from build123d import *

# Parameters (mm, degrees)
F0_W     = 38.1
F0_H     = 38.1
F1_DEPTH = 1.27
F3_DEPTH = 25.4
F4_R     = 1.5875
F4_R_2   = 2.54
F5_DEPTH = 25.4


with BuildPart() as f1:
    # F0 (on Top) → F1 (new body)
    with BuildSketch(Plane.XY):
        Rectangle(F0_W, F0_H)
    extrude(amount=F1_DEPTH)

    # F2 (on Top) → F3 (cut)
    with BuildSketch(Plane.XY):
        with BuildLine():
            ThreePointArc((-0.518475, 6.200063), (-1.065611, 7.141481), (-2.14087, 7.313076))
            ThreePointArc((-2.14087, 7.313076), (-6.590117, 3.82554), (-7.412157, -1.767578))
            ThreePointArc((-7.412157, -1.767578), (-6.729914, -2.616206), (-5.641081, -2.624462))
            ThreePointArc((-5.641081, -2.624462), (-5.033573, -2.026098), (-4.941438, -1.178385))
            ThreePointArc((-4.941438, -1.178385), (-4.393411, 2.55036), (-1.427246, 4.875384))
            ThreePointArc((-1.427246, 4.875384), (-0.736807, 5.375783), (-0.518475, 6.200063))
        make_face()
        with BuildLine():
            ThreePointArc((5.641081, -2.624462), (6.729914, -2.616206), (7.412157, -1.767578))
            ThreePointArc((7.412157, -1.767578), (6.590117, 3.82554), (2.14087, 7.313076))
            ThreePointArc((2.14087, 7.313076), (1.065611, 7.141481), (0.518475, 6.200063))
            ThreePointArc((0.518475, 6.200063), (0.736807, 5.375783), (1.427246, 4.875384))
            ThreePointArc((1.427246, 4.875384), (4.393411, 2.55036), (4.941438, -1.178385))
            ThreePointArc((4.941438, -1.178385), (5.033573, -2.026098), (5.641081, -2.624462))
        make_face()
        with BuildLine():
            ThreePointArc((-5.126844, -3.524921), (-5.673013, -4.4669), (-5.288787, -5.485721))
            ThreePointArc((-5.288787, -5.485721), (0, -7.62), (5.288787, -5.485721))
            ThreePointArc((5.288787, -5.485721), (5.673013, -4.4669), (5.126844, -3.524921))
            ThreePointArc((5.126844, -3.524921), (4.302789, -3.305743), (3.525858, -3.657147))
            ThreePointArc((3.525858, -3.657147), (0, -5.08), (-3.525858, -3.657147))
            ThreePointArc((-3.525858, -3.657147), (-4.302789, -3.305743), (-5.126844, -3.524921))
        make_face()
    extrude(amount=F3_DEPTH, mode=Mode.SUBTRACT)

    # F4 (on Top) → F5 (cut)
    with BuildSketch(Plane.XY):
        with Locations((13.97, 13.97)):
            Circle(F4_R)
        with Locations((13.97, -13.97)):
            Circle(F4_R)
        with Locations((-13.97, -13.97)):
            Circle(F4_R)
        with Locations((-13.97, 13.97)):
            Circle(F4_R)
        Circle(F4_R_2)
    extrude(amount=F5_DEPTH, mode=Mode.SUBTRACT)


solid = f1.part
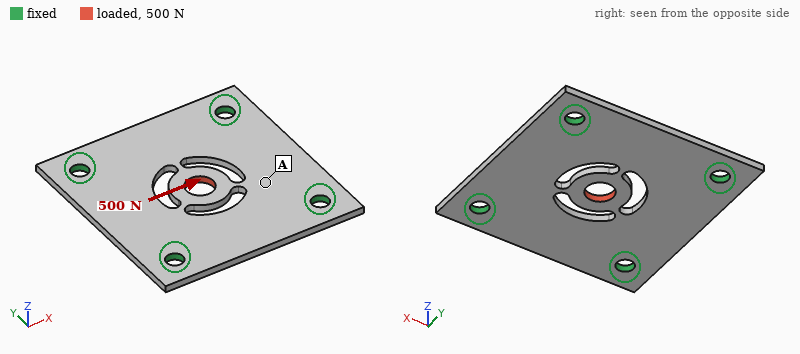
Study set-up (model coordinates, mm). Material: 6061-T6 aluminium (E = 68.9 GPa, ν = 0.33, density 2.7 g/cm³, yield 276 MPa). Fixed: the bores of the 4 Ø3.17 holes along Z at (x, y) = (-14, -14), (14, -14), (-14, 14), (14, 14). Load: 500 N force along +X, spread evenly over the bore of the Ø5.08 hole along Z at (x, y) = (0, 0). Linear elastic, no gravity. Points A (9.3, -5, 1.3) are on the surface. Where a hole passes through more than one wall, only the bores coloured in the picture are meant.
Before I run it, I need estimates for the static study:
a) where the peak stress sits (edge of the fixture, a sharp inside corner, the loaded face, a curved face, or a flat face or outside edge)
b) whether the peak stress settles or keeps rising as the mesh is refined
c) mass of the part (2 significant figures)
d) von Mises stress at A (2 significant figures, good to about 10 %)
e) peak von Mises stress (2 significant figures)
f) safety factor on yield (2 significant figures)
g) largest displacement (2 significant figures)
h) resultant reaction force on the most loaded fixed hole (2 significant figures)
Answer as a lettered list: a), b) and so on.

a) a curved face
b) settles
c) 4.5 g
d) 31 MPa
e) 280 MPa
f) 1.00
g) 26 µm
h) 170 N
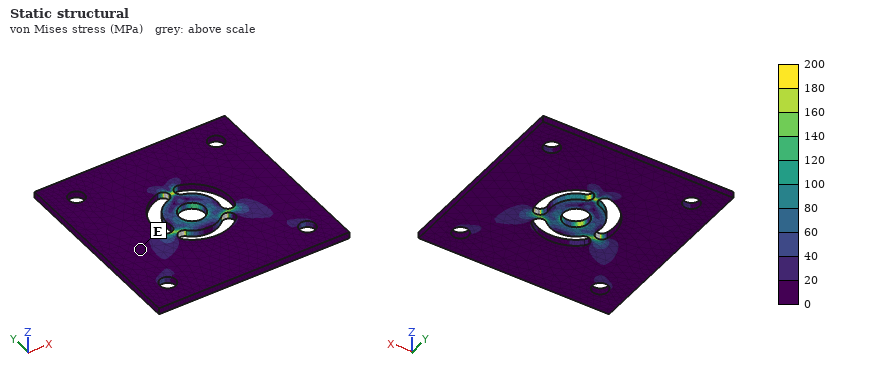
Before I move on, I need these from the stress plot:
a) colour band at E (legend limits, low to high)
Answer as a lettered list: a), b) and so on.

a) 0 to 20 MPa
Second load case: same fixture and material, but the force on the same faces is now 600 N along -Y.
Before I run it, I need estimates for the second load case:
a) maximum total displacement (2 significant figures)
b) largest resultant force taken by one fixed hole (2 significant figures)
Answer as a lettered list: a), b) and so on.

a) 34 µm
b) 180 N
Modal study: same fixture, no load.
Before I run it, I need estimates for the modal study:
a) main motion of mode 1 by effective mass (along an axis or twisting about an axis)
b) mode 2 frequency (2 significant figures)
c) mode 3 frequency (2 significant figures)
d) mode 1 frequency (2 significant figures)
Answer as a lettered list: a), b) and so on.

a) along Z
b) 9900 Hz
c) 9900 Hz
d) 6700 Hz
